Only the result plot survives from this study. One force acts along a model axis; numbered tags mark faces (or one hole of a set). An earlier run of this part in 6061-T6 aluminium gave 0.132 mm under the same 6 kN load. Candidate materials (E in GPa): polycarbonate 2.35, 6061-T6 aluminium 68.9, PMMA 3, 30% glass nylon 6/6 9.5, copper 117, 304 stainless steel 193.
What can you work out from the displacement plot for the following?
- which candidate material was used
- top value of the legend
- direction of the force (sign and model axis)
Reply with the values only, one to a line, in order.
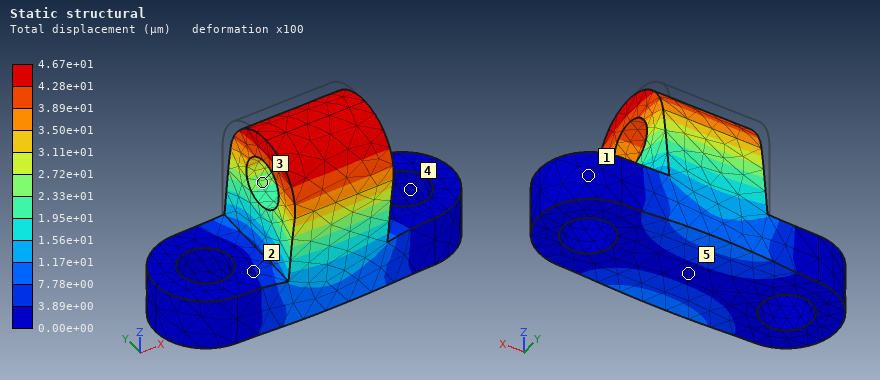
304 stainless steel
4.67e+01 µm
-Y
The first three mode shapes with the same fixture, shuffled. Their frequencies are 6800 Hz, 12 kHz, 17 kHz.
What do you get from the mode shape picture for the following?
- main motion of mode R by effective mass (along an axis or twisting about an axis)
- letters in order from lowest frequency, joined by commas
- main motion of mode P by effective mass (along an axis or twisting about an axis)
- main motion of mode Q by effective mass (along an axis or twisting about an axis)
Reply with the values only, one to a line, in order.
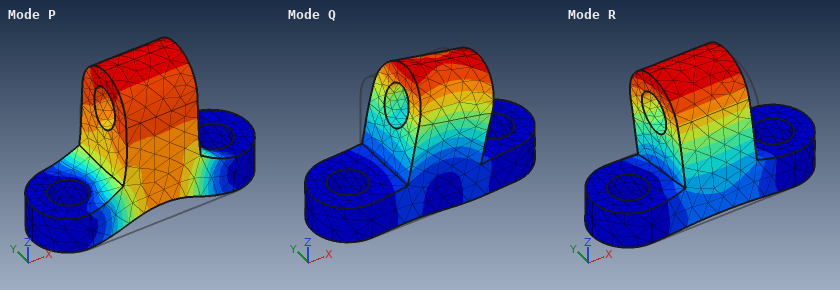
along Y
R, Q, P
along Z
along X
